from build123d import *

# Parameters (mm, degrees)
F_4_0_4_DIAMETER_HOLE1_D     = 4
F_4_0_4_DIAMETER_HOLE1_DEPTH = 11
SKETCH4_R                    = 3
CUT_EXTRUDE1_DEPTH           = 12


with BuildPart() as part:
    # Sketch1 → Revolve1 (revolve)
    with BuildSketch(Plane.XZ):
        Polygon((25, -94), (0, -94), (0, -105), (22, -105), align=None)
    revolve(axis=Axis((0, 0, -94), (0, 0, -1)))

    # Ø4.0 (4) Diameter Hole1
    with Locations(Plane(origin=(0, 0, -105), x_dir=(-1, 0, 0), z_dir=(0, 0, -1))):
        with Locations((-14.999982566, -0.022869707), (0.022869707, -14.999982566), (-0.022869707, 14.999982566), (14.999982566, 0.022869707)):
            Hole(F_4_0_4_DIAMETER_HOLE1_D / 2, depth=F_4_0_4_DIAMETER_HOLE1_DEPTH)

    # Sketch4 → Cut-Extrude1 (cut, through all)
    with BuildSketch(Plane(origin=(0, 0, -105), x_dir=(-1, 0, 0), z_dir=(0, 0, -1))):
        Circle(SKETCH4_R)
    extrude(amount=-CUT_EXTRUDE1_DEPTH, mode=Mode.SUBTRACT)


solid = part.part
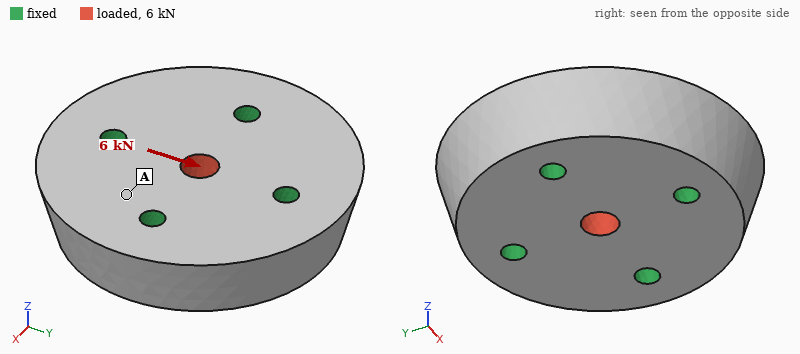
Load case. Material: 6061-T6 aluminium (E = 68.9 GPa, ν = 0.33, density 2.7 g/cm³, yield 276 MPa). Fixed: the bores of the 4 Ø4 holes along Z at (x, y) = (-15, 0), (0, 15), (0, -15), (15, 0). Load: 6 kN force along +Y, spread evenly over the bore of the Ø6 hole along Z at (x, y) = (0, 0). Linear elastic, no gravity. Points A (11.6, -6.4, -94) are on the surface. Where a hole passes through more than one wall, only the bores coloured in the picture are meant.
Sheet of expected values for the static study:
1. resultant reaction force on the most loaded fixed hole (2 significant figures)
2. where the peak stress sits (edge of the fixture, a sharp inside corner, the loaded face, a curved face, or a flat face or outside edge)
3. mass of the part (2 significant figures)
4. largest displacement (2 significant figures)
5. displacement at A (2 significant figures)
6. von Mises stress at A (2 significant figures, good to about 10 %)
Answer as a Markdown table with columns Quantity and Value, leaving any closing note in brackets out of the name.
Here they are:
| Quantity | Value |
|---|---|
| resultant reaction force on the most loaded fixed hole | 2.0 kN |
| where the peak stress sits | the loaded face |
| mass of the part | 49 g |
| largest displacement | 4.0 µm |
| displacement at A | 0.93 µm |
| von Mises stress at A | 5.6 MPa |
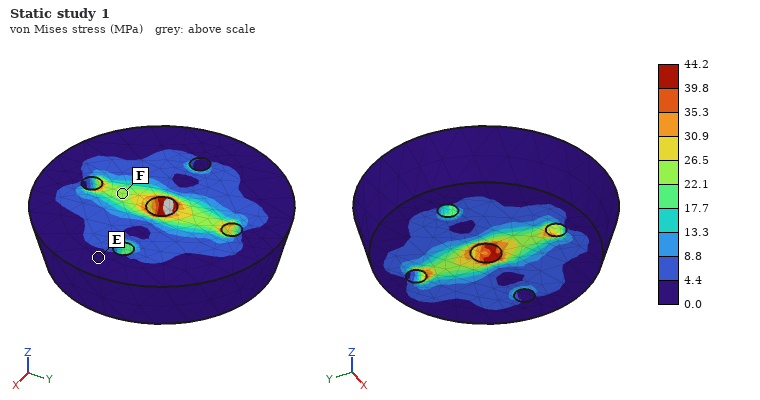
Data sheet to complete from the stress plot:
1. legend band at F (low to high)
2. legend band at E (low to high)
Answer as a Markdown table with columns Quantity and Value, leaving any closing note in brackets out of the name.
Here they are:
| Quantity | Value |
|---|---|
| legend band at F | 22.1 to 26.5 MPa |
| legend band at E | 0.0 to 4.4 MPa |
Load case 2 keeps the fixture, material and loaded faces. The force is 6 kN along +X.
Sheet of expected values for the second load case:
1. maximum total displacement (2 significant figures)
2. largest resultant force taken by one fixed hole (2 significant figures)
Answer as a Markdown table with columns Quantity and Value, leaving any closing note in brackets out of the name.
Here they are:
| Quantity | Value |
|---|---|
| maximum total displacement | 4.0 µm |
| largest resultant force taken by one fixed hole | 2.0 kN |
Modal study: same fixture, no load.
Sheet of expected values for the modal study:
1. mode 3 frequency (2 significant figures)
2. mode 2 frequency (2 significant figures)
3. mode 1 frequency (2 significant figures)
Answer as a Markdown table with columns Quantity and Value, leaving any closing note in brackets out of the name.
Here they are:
| Quantity | Value |
|---|---|
| mode 3 frequency | 39 kHz |
| mode 2 frequency | 39 kHz |
| mode 1 frequency | 37 kHz |
